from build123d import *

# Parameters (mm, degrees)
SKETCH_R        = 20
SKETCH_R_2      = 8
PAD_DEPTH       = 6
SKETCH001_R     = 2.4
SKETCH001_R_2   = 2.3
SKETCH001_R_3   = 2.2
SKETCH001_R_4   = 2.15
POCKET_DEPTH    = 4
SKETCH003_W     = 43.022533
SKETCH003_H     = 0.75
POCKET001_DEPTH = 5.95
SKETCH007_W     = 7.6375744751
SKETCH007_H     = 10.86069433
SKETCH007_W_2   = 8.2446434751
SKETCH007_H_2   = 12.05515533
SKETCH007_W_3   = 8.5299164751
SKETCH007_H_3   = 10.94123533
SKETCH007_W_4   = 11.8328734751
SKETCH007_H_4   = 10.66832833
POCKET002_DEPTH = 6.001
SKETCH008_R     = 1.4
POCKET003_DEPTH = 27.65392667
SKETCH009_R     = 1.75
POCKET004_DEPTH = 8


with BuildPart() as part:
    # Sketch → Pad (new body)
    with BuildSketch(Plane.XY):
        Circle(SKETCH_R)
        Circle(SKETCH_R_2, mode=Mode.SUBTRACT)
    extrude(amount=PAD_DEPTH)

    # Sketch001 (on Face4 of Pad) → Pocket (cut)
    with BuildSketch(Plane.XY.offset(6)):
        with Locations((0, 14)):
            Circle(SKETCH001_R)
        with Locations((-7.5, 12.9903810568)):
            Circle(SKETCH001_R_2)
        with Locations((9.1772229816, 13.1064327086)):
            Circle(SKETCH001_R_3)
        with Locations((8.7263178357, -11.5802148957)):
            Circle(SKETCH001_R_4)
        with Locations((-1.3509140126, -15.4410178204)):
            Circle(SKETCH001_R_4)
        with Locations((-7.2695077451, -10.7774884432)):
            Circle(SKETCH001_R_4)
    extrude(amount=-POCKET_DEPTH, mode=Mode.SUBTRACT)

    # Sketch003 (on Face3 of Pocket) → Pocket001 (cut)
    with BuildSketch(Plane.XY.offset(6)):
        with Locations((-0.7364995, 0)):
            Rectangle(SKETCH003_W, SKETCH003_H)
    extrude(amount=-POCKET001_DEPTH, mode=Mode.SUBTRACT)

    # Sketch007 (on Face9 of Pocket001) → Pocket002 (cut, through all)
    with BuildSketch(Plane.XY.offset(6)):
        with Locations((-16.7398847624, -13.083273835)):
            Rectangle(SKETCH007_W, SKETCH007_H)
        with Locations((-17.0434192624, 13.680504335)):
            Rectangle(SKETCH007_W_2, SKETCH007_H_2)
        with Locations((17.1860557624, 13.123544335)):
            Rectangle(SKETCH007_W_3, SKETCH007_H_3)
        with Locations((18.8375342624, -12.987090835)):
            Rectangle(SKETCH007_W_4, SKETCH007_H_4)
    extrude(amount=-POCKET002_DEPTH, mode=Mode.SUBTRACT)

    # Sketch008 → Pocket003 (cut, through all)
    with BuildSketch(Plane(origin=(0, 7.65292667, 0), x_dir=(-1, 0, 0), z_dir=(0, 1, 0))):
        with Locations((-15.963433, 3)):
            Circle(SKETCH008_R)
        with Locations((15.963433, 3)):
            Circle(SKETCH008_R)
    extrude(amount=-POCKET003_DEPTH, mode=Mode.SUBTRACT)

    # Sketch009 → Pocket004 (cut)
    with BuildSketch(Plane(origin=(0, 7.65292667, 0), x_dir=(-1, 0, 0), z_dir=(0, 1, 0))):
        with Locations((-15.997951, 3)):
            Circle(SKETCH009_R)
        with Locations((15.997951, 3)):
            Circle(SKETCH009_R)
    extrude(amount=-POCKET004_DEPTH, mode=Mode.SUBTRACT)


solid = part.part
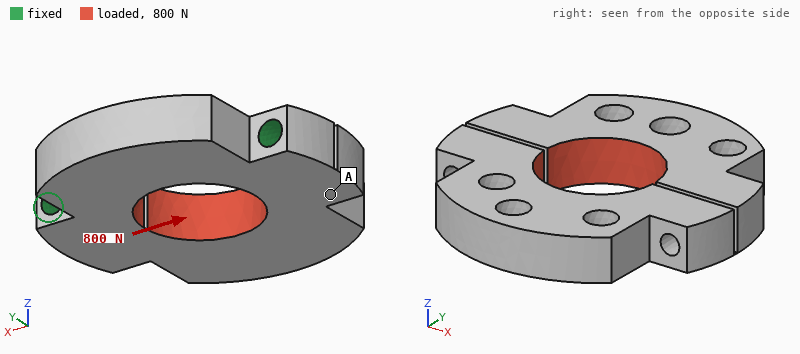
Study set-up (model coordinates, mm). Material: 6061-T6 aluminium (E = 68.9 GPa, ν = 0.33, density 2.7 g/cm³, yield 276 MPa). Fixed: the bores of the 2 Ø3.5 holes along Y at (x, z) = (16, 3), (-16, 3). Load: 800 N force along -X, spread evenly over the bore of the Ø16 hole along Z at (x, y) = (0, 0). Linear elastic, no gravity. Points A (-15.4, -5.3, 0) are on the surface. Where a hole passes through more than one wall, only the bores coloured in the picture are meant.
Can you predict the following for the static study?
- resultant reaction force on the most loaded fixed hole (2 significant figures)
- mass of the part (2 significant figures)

410 N
14 g
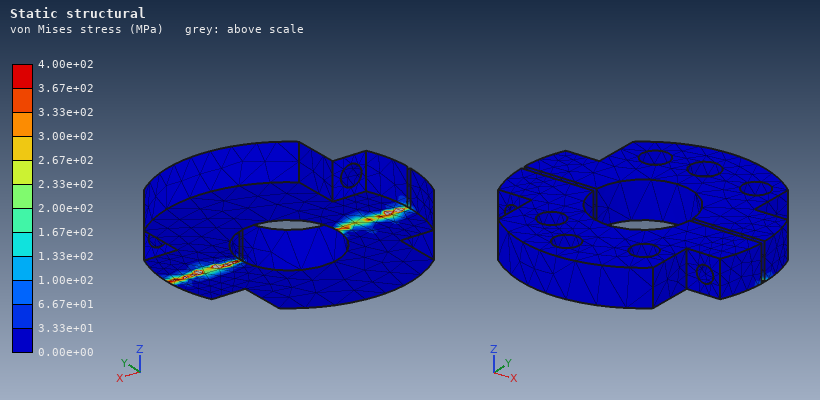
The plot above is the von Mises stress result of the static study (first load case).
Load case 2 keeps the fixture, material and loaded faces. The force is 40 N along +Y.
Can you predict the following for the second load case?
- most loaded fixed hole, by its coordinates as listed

(-16, 3)
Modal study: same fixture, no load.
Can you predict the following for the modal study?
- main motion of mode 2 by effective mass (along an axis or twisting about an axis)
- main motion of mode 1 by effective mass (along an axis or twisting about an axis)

along X
along Z
